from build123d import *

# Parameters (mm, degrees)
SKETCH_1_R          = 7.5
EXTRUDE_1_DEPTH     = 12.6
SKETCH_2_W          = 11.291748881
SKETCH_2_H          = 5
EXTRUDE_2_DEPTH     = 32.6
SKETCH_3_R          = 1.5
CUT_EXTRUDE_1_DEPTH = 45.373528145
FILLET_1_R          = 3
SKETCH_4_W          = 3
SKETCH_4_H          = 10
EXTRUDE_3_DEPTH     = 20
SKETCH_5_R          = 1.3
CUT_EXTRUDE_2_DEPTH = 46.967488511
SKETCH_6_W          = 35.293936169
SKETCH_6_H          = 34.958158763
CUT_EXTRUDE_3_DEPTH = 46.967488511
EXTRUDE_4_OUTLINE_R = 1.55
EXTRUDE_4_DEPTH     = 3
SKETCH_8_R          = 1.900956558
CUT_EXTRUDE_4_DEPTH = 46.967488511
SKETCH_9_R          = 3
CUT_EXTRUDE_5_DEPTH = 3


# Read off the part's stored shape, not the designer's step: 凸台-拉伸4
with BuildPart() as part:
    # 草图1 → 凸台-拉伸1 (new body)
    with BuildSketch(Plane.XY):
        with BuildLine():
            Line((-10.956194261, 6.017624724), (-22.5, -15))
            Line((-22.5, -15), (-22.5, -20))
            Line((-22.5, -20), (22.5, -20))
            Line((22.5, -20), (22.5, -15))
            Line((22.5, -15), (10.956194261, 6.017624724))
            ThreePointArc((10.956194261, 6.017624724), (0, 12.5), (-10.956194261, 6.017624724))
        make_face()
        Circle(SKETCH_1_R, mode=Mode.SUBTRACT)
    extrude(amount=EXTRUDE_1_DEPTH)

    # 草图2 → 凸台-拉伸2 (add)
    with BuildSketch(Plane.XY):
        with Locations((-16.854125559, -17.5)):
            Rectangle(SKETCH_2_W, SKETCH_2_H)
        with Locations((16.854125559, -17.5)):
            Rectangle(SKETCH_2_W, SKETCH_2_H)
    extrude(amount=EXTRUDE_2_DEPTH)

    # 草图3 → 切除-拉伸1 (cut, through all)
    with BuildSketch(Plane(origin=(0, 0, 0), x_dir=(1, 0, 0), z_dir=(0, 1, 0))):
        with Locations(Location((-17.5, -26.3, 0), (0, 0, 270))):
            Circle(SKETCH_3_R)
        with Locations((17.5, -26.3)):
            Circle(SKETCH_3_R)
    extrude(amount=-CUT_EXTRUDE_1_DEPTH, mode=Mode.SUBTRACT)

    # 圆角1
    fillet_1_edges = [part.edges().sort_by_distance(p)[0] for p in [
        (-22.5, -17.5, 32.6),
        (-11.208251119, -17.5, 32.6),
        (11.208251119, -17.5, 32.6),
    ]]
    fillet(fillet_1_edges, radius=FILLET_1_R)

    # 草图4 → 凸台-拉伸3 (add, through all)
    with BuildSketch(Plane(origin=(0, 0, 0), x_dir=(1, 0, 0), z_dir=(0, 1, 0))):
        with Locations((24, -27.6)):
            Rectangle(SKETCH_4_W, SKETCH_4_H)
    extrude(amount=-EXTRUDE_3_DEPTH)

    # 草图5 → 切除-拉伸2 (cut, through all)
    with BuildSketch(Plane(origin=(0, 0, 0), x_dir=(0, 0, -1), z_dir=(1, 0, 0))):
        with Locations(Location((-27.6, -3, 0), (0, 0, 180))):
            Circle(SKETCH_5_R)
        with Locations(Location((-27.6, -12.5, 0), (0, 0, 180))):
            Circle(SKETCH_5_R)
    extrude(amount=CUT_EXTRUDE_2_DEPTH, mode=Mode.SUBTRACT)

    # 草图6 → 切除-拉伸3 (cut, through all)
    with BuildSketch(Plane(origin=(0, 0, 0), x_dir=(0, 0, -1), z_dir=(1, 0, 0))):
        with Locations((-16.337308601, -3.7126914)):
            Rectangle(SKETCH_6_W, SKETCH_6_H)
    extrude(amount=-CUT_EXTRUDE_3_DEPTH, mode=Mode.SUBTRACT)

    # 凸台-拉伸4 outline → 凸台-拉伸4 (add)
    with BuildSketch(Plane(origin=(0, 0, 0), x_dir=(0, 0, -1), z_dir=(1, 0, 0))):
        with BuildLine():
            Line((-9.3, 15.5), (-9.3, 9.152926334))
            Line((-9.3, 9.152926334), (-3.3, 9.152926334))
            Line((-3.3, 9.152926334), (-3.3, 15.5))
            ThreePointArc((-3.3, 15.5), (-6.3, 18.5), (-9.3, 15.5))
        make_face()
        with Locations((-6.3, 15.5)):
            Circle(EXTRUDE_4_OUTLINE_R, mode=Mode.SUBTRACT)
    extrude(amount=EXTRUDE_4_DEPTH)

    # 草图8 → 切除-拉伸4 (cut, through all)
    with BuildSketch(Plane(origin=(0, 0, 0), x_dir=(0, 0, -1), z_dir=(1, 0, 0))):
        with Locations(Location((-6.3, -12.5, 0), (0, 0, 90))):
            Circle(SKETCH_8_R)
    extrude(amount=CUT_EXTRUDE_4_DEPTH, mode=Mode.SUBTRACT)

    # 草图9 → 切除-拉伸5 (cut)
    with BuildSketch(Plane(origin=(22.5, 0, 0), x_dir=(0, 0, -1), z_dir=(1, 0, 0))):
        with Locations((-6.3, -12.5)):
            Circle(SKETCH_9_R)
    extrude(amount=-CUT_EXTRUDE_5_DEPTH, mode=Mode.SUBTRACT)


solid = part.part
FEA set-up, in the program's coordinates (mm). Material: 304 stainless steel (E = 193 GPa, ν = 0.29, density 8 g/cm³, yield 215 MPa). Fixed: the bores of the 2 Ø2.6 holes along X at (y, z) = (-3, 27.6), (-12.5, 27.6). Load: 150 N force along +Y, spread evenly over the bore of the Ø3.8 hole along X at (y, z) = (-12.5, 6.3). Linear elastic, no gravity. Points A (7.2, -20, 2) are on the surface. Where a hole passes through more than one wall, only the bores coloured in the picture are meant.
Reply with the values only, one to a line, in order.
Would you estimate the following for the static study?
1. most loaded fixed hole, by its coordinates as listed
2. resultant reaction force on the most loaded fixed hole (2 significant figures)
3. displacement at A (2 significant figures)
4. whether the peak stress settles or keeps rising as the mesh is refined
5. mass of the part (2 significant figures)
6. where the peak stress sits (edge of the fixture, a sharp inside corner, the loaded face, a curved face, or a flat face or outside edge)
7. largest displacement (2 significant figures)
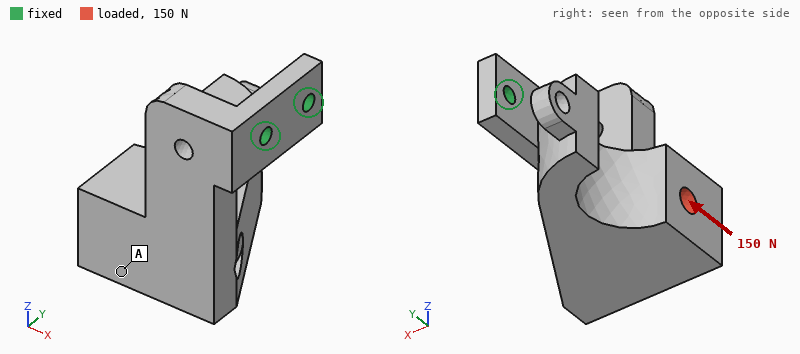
(-12.5, 27.6)
240 N
0.095 mm
keeps rising
55 g
edge of the fixture
0.17 mm
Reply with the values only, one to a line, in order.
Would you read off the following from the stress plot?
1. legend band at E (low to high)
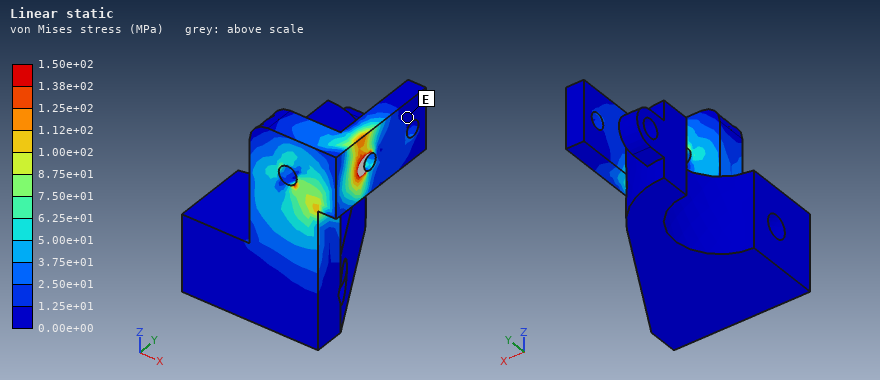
0.00e+00 to 1.25e+01 MPa
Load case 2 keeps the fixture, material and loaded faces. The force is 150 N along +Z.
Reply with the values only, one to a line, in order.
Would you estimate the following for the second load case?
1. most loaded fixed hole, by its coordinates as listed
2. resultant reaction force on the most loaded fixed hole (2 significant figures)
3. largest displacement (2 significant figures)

(-12.5, 27.6)
140 N
68 µm
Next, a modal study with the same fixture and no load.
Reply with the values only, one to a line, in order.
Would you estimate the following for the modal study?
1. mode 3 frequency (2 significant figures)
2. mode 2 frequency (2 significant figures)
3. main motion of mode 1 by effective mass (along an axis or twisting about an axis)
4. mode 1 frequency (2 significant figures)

2400 Hz
1000 Hz
along Y
900 Hz
